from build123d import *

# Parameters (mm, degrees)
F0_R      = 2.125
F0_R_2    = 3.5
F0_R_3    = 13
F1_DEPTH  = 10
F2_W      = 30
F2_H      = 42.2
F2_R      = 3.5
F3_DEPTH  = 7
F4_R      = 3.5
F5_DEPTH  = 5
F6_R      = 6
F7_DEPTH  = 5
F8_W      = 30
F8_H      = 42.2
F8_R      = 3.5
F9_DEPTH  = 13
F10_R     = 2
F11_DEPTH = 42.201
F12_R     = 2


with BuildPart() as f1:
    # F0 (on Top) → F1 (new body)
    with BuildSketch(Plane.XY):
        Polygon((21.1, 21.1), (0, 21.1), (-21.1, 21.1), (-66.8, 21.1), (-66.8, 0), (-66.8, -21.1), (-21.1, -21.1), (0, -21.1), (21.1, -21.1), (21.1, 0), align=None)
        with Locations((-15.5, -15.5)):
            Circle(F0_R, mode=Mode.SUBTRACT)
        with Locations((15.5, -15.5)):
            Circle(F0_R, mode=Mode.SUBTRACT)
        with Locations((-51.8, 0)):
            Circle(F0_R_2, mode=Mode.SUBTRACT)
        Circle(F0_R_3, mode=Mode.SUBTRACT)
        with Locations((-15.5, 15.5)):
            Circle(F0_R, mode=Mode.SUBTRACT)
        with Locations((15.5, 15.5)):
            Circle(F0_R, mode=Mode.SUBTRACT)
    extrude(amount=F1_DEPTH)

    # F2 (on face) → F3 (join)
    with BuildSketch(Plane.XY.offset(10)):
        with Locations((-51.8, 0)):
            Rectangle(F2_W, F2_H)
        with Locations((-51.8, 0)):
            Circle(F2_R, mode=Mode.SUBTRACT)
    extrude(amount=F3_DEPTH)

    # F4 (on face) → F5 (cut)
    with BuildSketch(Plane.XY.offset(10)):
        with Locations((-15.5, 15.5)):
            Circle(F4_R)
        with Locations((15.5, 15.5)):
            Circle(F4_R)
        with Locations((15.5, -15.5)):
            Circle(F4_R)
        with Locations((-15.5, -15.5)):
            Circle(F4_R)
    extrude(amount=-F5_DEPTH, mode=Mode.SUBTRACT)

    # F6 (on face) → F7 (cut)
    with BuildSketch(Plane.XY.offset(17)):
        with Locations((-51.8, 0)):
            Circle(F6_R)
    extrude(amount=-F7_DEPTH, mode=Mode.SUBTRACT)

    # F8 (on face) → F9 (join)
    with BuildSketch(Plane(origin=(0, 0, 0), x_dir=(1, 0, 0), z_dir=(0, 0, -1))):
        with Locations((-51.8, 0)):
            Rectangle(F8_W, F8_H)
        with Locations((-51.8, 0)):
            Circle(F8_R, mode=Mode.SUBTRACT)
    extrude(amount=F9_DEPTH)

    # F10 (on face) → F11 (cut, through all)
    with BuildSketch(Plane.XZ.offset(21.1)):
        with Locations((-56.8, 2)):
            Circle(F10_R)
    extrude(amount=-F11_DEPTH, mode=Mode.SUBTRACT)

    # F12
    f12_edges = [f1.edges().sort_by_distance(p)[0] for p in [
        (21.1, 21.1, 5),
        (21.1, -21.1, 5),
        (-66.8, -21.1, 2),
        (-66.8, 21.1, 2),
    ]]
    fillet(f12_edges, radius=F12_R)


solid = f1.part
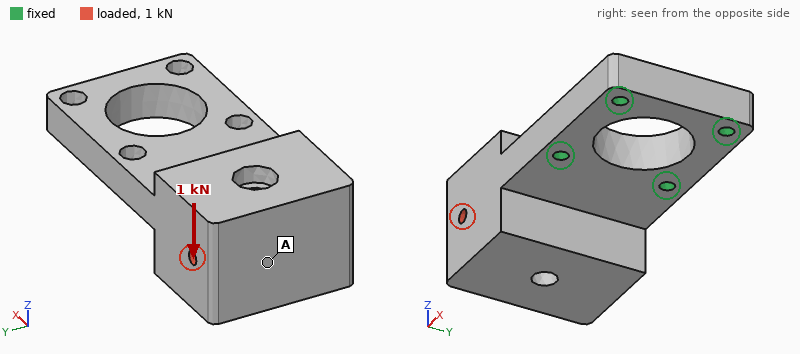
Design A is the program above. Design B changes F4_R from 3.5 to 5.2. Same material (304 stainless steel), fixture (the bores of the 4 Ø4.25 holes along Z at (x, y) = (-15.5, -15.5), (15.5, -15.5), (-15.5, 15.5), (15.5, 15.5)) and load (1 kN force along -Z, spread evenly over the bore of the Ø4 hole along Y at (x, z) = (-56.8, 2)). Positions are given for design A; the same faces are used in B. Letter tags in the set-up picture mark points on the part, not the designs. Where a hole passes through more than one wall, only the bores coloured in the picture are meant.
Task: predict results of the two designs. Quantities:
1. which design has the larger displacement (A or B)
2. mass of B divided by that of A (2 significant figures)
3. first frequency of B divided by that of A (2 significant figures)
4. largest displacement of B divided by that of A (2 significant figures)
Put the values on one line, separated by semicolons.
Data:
B; 0.98; 0.91; 1.2
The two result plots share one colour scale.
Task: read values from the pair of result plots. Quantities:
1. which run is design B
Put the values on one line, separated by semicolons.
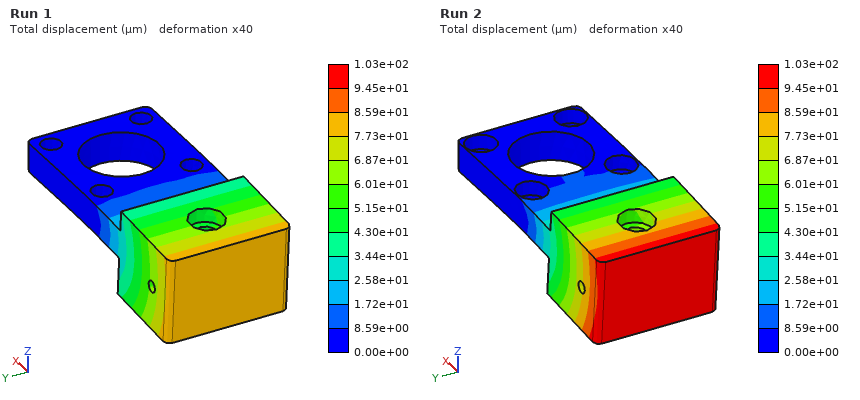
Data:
Run 2
